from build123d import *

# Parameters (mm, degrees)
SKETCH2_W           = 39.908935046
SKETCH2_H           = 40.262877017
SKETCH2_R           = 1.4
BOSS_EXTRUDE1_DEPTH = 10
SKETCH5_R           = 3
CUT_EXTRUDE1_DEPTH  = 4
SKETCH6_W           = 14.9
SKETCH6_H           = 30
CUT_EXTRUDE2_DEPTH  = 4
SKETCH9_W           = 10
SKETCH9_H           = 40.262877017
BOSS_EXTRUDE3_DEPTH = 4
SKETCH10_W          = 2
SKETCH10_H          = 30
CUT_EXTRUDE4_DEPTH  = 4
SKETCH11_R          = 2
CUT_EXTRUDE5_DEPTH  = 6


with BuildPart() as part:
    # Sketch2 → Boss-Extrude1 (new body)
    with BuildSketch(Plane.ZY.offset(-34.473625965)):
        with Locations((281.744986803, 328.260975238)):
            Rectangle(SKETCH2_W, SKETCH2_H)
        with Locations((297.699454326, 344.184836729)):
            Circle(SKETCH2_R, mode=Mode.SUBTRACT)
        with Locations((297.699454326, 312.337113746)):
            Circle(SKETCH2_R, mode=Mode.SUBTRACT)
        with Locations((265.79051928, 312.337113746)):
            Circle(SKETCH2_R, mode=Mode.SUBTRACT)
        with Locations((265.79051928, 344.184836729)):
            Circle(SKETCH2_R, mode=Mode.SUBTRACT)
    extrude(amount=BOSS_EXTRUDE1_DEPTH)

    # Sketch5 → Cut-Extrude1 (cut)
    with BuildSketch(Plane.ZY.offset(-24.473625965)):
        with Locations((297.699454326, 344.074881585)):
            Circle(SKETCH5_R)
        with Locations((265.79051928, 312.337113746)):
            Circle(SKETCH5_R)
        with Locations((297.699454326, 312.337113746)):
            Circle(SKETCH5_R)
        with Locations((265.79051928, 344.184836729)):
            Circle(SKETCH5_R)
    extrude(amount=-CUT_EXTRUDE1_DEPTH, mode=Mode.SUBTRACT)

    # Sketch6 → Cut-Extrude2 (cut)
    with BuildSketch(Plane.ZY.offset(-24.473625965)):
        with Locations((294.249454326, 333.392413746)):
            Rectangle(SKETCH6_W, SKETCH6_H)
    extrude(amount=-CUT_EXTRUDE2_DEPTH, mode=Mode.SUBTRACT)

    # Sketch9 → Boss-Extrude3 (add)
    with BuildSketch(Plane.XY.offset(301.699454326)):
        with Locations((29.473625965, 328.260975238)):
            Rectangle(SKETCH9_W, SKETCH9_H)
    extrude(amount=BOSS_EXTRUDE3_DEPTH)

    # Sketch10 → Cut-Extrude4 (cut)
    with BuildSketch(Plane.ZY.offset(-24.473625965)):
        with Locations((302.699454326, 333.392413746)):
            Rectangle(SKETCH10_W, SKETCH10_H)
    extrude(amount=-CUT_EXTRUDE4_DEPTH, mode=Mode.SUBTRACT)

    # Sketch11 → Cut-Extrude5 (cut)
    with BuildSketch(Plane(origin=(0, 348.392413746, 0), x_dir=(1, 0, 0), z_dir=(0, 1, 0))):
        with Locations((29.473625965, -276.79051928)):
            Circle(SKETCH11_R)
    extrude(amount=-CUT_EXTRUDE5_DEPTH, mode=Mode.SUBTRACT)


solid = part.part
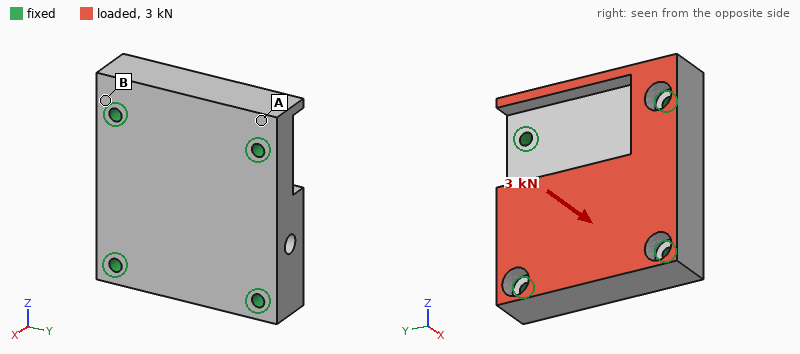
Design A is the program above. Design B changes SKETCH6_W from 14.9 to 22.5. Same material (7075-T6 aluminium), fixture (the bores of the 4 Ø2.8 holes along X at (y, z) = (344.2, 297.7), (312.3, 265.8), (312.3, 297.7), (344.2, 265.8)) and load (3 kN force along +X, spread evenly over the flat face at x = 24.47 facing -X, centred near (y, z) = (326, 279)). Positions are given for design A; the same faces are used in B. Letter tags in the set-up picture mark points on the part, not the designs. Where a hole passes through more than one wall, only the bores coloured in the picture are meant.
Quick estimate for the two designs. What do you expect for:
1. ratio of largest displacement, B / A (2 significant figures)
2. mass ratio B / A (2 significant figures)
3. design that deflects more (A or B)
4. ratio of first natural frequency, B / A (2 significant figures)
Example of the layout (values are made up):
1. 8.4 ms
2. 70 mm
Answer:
1. 1.1
2. 0.97
3. B
4. 0.98
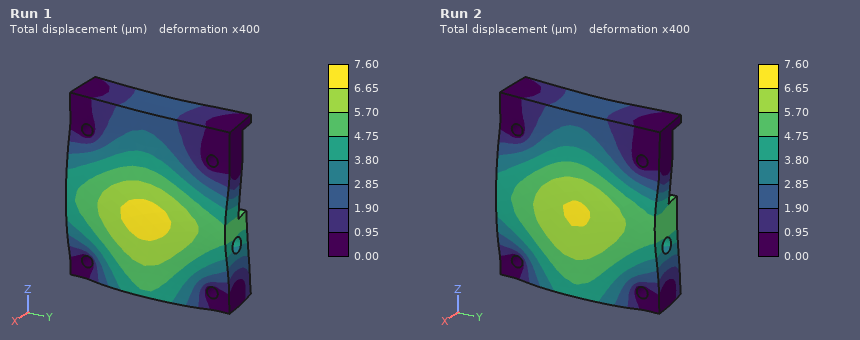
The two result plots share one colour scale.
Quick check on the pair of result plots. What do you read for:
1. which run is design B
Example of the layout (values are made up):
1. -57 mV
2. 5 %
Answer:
1. Run 1
